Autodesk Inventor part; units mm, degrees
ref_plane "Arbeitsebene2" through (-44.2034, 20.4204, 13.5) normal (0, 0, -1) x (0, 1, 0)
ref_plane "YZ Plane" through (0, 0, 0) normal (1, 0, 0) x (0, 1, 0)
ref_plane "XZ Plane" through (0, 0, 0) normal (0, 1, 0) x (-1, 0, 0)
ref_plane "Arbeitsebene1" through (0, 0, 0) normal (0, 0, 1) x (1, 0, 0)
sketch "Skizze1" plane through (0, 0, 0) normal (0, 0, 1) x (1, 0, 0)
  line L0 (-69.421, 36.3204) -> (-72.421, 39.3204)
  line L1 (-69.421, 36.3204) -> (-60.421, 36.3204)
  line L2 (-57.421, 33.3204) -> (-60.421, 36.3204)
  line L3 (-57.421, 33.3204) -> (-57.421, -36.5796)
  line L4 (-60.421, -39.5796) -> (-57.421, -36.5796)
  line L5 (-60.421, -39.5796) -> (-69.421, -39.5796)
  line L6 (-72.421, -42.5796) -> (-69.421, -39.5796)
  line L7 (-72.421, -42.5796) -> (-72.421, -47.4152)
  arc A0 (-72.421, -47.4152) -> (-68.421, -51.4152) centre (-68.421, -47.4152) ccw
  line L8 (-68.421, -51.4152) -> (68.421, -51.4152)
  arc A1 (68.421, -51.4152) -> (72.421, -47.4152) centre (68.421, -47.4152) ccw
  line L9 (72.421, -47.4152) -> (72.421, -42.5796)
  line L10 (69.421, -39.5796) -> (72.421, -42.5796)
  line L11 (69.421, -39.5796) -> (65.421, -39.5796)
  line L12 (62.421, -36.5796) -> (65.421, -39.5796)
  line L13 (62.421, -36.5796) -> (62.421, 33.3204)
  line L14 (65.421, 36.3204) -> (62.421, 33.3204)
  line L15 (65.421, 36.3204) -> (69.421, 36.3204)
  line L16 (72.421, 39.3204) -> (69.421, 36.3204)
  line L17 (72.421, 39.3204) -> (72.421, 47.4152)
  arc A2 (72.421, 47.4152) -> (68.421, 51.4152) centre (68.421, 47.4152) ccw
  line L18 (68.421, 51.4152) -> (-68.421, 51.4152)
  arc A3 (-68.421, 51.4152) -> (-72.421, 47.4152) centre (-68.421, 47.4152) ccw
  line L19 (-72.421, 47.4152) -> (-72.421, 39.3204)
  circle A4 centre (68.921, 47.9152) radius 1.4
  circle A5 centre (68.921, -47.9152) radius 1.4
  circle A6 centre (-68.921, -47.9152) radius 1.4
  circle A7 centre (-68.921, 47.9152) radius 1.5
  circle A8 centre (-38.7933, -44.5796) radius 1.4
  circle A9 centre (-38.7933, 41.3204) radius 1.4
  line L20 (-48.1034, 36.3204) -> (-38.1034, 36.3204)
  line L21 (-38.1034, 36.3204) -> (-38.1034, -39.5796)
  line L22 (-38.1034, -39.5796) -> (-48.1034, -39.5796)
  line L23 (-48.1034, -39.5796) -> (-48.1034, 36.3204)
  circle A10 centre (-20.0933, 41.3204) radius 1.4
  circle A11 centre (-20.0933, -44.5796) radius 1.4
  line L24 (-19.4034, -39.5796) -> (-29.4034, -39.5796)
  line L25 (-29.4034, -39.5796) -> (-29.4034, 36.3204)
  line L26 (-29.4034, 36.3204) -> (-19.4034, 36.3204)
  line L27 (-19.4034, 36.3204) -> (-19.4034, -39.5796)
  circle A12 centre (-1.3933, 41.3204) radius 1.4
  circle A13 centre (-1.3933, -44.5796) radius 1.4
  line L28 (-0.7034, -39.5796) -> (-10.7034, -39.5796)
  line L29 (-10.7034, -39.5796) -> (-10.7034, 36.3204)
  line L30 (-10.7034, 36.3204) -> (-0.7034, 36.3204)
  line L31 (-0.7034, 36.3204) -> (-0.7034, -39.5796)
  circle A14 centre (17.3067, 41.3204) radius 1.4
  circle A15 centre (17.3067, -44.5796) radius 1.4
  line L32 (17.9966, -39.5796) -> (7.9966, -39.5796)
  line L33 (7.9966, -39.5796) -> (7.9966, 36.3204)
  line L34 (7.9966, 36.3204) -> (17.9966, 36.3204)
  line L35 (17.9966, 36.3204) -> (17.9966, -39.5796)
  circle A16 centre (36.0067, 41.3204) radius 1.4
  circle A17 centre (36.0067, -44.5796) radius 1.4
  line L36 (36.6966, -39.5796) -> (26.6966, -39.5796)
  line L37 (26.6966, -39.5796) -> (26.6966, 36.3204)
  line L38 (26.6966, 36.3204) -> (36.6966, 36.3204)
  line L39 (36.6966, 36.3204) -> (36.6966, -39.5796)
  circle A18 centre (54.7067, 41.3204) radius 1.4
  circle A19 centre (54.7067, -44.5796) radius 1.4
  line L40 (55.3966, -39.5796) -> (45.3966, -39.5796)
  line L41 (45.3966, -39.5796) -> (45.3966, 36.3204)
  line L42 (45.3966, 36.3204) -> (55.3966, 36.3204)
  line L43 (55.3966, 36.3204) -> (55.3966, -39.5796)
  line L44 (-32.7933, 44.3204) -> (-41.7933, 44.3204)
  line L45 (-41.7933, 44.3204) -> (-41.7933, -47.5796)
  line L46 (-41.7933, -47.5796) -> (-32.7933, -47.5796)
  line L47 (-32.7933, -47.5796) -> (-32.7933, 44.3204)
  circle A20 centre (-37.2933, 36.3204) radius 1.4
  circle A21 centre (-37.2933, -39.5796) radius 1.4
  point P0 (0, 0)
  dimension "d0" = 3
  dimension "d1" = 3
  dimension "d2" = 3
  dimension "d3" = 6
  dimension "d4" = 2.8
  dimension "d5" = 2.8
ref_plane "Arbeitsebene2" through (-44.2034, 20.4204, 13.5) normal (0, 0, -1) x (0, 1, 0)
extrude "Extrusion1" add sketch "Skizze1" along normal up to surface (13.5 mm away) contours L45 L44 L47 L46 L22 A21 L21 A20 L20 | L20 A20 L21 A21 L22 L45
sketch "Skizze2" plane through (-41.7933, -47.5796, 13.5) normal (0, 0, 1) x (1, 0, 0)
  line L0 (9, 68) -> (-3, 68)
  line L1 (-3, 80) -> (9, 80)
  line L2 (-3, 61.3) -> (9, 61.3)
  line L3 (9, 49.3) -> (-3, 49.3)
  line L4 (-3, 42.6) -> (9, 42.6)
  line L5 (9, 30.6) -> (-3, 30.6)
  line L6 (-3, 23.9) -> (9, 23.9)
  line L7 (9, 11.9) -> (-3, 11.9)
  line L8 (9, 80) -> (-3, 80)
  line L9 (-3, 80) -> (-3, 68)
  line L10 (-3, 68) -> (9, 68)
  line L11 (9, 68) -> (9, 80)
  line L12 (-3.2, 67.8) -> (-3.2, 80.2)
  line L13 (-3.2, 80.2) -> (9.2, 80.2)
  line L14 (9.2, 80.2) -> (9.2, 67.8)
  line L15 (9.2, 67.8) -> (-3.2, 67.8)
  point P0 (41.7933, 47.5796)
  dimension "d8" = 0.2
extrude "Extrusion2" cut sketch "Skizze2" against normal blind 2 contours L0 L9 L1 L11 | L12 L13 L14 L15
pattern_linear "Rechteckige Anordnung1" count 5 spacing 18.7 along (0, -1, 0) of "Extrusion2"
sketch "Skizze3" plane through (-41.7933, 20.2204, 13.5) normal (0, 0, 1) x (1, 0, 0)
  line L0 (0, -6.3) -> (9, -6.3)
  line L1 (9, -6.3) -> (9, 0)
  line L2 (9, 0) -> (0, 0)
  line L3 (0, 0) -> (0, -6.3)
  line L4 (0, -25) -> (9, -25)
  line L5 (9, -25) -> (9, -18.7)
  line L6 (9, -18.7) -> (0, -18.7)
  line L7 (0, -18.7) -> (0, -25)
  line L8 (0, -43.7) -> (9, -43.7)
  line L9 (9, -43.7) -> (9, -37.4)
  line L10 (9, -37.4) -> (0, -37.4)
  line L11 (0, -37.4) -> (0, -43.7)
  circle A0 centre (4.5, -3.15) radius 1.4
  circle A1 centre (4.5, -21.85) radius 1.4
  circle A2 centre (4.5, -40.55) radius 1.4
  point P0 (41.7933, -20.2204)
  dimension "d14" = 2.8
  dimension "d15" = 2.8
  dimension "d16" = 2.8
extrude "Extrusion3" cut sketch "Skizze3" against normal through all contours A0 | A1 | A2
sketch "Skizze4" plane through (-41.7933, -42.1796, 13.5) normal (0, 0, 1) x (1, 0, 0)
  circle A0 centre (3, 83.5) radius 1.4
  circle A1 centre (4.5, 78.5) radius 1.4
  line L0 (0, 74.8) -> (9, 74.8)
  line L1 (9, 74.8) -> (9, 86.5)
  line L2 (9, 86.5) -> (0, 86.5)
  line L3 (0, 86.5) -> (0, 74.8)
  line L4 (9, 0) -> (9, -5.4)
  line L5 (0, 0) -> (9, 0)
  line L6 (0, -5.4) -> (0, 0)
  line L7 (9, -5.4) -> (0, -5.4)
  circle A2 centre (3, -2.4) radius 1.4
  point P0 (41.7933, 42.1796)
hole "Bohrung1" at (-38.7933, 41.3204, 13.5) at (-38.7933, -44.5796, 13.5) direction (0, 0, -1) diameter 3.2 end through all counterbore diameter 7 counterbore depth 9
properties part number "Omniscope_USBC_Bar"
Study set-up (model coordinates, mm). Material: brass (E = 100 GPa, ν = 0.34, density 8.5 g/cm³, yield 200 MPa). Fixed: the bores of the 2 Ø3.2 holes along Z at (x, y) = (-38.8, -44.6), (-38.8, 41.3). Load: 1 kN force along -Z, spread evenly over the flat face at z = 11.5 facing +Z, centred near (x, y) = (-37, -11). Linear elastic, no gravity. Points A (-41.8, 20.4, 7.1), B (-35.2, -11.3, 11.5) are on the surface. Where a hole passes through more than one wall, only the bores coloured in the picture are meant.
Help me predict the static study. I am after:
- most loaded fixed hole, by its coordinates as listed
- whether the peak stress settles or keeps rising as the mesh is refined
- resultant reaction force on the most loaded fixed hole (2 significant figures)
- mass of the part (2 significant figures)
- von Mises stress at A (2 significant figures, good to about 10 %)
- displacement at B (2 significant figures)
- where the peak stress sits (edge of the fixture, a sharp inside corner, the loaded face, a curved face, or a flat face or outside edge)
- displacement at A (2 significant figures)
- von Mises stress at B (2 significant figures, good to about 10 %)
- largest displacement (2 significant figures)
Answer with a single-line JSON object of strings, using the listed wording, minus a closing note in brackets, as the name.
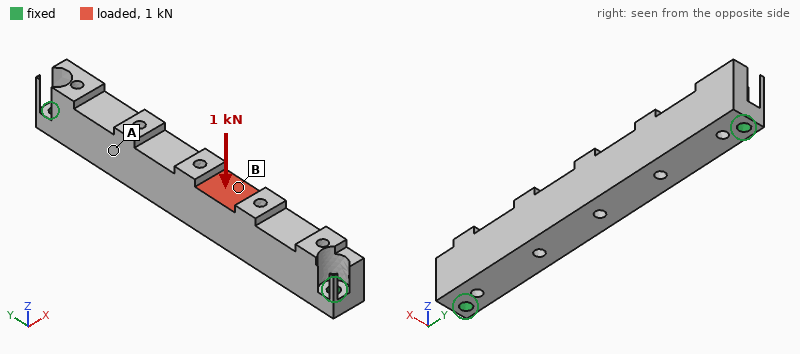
{"most loaded fixed hole, by its coordinates as listed": "(-38.8, -44.6)", "whether the peak stress settles or keeps rising as the mesh is refined": "keeps rising", "resultant reaction force on the most loaded fixed hole": "1.1 kN", "mass of the part": "77 g", "von Mises stress at A": "17 MPa", "displacement at B": "58 µm", "where the peak stress sits": "edge of the fixture", "displacement at A": "30 µm", "von Mises stress at B": "65 MPa", "largest displacement": "61 µm"}
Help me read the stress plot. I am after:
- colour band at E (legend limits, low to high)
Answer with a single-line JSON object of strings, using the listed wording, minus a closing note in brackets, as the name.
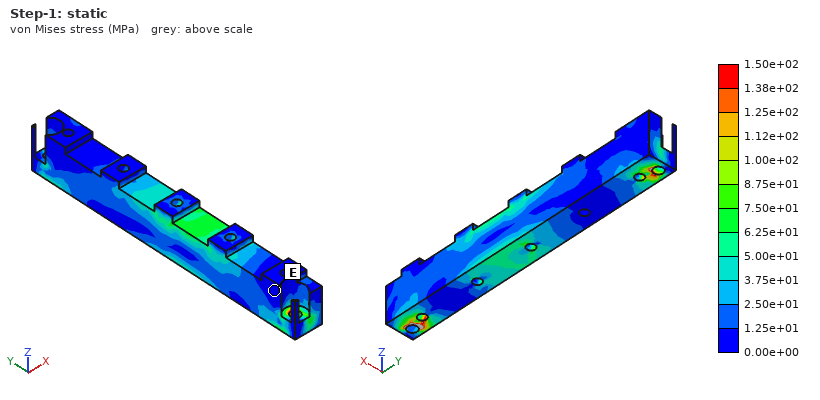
{"colour band at E": "0.00e+00 to 1.25e+01 MPa"}
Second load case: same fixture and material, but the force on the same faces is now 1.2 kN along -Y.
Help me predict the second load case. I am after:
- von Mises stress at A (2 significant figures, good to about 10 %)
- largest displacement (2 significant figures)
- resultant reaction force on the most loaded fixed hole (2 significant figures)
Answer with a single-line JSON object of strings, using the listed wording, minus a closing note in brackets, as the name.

{"von Mises stress at A": "9.2 MPa", "largest displacement": "8.8 µm", "resultant reaction force on the most loaded fixed hole": "610 N"}
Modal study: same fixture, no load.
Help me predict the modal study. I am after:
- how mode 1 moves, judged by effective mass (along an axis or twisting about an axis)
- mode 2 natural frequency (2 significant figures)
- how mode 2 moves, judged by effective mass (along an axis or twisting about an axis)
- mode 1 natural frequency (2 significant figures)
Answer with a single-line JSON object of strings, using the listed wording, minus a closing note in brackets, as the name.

{"how mode 1 moves, judged by effective mass": "along X", "mode 2 natural frequency": "3500 Hz", "how mode 2 moves, judged by effective mass": "along Z", "mode 1 natural frequency": "2700 Hz"}
